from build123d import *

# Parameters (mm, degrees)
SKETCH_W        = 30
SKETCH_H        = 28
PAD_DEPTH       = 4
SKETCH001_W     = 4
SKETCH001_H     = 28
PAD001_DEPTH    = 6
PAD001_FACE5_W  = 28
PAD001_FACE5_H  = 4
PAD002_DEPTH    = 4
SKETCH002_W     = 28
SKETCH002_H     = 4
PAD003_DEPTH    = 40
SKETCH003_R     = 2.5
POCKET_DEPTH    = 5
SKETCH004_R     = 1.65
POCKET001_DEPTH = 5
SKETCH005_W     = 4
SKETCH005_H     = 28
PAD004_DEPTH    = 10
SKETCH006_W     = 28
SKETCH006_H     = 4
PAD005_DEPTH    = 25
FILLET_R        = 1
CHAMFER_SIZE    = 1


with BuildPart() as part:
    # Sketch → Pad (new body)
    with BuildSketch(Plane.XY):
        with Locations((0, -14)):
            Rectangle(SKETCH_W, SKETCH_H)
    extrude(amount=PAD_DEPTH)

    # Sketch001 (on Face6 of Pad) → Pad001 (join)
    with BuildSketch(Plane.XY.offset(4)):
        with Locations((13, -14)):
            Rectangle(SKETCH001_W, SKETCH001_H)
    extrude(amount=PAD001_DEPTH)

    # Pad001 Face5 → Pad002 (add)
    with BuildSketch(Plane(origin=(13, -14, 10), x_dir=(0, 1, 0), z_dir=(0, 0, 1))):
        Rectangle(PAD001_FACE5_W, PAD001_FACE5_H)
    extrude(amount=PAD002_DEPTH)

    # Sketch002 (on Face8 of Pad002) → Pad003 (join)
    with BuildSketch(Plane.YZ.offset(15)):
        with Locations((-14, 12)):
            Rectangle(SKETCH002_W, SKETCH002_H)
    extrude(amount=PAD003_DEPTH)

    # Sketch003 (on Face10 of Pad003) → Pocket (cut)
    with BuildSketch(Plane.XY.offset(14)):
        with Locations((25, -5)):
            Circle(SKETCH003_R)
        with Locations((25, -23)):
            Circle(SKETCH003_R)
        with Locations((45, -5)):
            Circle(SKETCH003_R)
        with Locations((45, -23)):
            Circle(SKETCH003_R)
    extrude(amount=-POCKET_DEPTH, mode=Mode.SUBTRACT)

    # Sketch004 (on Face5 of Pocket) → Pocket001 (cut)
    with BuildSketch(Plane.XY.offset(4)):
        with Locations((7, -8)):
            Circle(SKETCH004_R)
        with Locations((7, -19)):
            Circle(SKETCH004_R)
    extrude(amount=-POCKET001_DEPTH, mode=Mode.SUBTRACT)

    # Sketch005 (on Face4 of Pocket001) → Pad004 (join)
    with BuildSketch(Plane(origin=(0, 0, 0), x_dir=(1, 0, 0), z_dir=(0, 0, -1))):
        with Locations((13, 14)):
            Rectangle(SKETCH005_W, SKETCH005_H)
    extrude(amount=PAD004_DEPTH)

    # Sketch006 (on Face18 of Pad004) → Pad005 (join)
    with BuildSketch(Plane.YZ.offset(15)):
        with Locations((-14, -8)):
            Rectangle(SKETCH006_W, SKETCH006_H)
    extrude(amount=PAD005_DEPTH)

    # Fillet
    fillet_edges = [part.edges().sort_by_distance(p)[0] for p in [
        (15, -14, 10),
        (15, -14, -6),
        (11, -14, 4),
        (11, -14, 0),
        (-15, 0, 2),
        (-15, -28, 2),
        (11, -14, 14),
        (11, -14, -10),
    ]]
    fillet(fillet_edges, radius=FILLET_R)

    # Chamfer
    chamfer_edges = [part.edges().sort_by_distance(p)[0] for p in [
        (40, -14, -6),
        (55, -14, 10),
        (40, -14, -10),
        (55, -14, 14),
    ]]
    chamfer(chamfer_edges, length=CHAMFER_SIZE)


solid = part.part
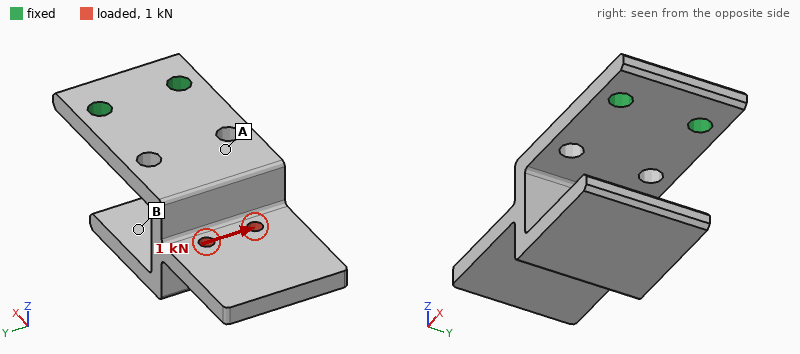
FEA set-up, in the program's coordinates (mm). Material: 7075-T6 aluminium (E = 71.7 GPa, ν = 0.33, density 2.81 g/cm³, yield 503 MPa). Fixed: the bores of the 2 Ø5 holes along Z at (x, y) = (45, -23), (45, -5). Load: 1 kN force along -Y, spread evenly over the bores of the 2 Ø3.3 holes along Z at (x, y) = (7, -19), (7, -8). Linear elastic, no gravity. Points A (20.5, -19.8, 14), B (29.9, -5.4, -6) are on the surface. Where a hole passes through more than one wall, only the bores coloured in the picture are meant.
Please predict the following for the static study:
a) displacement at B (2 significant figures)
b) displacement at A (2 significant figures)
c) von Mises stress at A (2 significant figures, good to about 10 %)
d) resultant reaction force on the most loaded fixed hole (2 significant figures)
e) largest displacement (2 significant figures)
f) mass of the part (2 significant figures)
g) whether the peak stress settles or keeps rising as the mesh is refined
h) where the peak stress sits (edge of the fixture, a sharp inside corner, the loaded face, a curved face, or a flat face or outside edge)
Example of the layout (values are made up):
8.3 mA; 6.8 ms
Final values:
0.29 mm; 0.066 mm; 66 MPa; 2.0 kN; 0.40 mm; 35 g; keeps rising; edge of the fixture
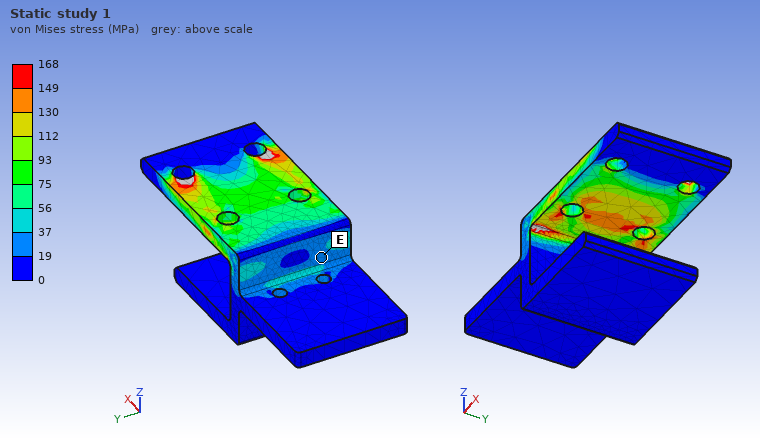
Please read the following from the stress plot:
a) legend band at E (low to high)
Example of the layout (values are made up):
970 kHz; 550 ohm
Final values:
19 to 37 MPa
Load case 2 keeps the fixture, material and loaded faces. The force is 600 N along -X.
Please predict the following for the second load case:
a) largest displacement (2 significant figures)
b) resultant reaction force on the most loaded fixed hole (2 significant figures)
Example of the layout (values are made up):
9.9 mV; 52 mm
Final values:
0.88 mm; 320 N
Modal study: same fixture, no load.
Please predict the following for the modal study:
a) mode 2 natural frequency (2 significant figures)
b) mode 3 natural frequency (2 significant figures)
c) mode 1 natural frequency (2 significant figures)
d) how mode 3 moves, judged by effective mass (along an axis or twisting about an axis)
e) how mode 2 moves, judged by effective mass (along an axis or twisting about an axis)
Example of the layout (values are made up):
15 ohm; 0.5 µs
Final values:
1500 Hz; 1900 Hz; 690 Hz; along Z; along Y
